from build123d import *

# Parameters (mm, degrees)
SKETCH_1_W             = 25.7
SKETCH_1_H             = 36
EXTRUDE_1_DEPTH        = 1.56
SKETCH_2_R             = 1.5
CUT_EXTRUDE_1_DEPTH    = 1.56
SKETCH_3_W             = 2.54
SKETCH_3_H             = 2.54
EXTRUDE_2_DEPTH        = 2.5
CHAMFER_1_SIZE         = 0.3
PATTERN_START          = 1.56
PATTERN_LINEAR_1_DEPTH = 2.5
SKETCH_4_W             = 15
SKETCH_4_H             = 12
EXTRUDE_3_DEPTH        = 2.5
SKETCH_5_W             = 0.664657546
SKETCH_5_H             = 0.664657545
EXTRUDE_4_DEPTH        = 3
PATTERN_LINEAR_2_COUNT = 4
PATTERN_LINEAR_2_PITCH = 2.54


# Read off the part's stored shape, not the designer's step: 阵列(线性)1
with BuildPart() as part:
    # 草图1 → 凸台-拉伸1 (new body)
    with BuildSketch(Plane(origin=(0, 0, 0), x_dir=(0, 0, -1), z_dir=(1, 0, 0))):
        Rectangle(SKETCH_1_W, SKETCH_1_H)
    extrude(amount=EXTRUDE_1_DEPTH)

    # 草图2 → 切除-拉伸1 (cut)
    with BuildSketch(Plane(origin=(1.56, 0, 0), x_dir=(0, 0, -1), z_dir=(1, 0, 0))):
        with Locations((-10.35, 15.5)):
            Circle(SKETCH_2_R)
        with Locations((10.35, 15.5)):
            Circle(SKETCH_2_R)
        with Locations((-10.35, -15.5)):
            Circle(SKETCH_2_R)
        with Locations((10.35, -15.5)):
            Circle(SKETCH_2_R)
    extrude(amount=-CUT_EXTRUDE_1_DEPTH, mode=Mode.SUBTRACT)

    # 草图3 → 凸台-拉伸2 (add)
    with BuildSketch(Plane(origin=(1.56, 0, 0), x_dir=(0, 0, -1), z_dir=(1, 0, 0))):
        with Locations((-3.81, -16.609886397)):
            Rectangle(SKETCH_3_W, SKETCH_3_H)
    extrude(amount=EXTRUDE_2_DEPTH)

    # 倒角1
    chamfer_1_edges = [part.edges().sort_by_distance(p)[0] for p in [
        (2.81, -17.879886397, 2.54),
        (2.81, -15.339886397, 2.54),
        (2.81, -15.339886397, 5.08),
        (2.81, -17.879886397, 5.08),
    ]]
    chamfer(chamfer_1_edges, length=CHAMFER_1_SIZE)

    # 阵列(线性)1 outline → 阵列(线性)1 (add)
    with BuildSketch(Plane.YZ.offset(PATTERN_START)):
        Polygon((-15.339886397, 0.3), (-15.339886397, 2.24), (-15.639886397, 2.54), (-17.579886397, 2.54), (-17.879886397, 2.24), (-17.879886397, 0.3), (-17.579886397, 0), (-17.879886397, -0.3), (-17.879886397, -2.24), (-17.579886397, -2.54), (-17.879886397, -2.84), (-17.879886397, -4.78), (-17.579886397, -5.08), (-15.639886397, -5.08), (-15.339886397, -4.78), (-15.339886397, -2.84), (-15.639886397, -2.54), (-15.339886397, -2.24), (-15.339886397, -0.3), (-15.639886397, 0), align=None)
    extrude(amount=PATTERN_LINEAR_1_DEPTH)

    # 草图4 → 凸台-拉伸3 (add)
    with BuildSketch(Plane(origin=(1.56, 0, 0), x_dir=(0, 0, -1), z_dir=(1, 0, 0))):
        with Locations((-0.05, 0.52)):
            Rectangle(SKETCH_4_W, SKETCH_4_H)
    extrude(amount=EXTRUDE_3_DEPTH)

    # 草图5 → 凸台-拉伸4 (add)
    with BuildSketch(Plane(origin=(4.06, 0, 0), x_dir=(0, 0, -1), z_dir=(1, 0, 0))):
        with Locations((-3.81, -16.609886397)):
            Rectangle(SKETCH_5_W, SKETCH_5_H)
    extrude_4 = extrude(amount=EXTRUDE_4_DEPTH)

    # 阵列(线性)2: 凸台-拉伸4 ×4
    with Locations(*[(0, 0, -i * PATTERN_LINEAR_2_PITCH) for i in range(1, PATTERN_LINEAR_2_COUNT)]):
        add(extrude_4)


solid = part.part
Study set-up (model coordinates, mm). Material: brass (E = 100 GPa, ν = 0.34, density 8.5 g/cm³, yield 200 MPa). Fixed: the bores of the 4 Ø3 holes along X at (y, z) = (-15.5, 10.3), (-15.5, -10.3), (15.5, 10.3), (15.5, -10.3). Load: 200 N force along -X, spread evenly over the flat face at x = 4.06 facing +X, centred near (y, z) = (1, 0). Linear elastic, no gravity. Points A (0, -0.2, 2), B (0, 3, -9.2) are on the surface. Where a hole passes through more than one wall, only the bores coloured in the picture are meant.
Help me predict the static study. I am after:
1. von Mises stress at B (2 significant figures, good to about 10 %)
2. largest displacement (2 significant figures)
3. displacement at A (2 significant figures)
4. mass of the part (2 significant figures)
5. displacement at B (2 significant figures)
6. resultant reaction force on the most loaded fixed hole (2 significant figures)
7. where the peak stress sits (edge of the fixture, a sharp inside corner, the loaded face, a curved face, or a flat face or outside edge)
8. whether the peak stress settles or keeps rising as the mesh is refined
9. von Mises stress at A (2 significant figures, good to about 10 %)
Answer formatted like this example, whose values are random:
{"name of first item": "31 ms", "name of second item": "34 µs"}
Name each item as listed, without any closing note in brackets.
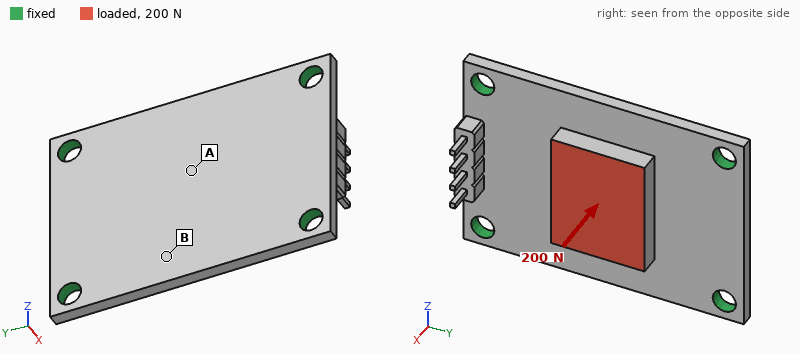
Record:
{"von Mises stress at B": "18 MPa", "largest displacement": "17 µm", "displacement at A": "17 µm", "mass of the part": "16 g", "displacement at B": "16 µm", "resultant reaction force on the most loaded fixed hole": "60 N", "where the peak stress sits": "edge of the fixture", "whether the peak stress settles or keeps rising as the mesh is refined": "keeps rising", "von Mises stress at A": "9.6 MPa"}
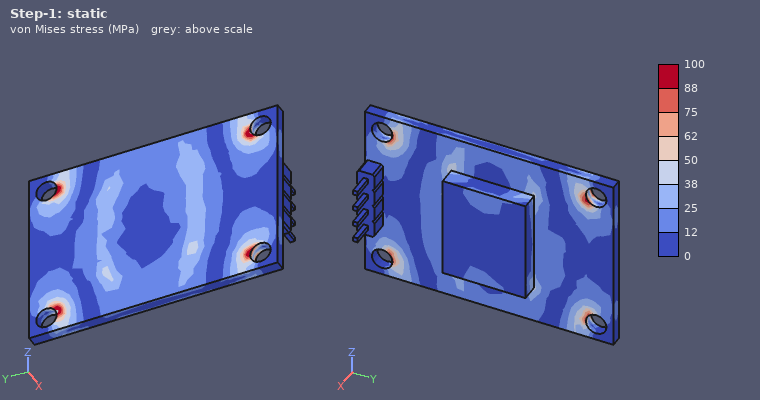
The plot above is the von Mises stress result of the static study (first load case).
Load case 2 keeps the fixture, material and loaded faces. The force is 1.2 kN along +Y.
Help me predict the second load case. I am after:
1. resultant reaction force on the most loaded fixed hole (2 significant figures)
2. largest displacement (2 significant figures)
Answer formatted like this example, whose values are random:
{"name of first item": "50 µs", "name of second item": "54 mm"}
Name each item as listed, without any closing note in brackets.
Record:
{"resultant reaction force on the most loaded fixed hole": "340 N", "largest displacement": "21 µm"}
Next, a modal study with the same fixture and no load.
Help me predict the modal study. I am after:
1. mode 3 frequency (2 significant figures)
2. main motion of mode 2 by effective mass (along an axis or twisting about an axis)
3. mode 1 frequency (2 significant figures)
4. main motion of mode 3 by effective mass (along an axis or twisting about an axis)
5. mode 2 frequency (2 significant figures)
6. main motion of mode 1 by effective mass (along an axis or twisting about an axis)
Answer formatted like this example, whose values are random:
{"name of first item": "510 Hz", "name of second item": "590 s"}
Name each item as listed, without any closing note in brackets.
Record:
{"mode 3 frequency": "13 kHz", "main motion of mode 2 by effective mass": "twisting about Y", "mode 1 frequency": "5500 Hz", "main motion of mode 3 by effective mass": "twisting about Z", "mode 2 frequency": "8100 Hz", "main motion of mode 1 by effective mass": "along X"}
